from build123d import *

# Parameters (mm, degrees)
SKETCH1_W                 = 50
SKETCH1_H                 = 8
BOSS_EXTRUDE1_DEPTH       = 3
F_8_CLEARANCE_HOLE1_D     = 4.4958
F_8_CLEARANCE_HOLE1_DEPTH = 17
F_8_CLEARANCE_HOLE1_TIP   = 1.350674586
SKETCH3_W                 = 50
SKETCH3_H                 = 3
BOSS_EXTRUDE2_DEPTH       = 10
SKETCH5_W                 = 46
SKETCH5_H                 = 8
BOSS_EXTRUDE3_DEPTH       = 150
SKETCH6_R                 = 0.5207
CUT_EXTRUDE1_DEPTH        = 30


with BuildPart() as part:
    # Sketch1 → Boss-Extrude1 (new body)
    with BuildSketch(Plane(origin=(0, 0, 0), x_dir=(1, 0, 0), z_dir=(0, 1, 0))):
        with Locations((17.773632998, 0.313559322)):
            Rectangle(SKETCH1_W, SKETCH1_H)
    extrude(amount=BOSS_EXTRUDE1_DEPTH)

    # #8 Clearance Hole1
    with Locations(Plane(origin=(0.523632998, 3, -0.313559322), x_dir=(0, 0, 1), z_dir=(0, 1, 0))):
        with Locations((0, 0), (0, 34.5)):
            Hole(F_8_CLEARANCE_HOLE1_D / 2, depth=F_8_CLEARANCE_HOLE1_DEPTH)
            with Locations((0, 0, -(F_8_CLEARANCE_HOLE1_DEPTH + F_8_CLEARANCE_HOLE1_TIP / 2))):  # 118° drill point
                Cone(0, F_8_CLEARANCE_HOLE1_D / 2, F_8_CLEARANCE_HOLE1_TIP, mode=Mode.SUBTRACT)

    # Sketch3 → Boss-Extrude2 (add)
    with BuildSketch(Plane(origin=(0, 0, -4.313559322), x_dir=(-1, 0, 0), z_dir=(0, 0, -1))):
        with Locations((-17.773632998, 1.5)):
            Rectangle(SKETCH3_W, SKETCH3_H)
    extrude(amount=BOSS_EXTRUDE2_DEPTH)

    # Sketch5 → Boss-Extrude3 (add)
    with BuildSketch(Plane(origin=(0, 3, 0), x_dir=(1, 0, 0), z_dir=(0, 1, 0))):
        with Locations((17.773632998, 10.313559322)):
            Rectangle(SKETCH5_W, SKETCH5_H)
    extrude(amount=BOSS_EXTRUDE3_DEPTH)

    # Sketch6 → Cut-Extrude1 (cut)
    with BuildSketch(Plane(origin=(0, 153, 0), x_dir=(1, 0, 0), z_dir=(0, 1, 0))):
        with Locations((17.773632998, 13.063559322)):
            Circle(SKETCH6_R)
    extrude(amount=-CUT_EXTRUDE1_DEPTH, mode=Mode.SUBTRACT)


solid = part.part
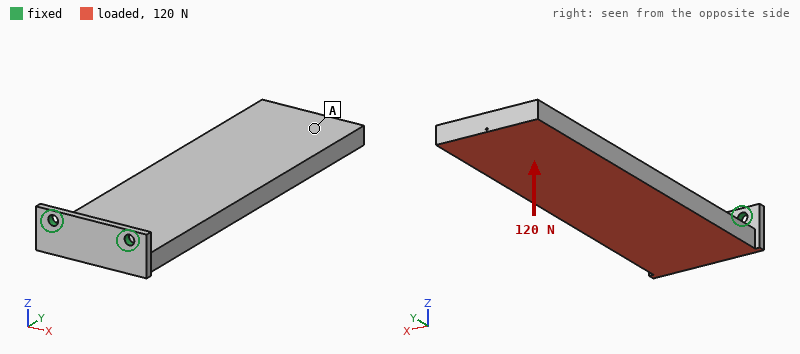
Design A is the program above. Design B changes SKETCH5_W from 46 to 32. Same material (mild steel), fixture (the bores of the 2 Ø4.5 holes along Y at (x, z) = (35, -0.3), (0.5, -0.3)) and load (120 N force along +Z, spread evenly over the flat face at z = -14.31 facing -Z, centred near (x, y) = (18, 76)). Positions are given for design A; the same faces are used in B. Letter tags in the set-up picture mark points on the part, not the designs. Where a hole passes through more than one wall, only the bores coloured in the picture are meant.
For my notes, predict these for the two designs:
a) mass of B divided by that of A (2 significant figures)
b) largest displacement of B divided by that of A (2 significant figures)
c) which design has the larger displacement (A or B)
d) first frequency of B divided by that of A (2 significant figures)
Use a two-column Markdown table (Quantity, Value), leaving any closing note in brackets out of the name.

| Quantity | Value |
|---|---|
| mass of B divided by that of A | 0.71 |
| largest displacement of B divided by that of A | 1.2 |
| which design has the larger displacement | B |
| first frequency of B divided by that of A | 1.1 |
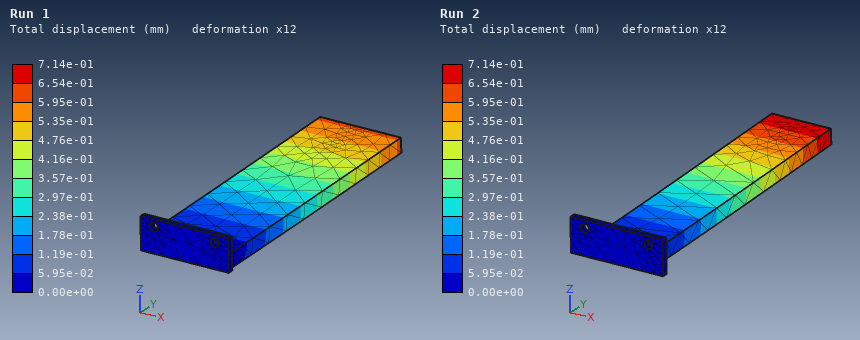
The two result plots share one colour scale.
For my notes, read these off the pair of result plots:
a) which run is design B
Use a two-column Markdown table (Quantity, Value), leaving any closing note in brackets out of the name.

| Quantity | Value |
|---|---|
| which run is design B | Run 2 |
